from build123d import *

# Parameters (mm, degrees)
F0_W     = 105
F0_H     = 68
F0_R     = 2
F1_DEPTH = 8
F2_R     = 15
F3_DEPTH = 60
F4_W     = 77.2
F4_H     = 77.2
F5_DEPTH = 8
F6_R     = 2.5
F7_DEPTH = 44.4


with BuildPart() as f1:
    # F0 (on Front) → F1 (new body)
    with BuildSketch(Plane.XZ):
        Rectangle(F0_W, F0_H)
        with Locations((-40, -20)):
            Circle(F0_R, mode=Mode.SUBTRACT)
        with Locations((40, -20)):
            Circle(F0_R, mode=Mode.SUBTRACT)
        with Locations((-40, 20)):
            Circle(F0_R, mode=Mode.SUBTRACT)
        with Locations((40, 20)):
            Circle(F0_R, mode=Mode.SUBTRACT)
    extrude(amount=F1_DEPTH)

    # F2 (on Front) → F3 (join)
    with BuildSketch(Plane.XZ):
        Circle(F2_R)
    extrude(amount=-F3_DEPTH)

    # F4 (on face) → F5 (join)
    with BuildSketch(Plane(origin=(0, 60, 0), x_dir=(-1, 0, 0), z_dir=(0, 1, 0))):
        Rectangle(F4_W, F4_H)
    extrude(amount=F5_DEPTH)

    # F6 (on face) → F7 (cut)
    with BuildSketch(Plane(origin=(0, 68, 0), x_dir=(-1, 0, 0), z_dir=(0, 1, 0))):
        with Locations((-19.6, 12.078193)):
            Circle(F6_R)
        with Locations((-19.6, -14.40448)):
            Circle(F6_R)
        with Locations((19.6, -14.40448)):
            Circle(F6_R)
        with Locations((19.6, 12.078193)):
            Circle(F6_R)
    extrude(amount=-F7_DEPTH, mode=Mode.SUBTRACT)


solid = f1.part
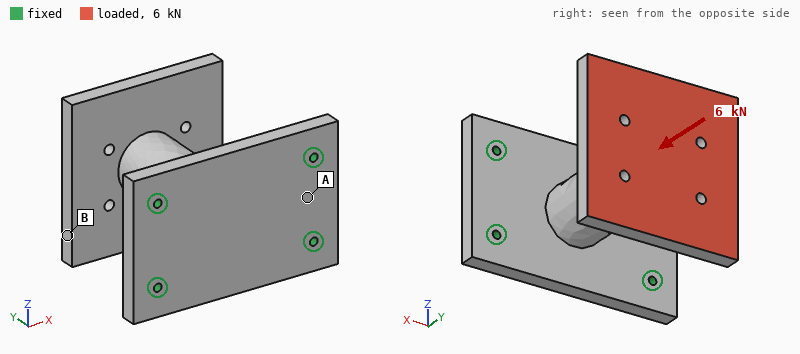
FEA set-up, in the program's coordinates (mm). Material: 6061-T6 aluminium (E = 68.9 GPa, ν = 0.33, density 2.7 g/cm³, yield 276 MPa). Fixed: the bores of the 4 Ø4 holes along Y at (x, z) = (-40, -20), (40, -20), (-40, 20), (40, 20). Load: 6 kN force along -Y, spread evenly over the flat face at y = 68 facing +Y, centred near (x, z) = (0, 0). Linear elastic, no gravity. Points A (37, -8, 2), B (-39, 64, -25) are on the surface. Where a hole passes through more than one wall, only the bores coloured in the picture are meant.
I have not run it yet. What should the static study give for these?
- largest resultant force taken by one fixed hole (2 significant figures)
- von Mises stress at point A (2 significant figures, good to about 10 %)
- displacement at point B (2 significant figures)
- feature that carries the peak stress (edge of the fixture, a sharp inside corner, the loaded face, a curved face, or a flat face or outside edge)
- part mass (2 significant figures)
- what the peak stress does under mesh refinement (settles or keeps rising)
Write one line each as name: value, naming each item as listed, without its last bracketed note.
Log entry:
largest resultant force taken by one fixed hole: 1.6 kN
von Mises stress at point A: 23 MPa
displacement at point B: 0.14 mm
feature that carries the peak stress: edge of the fixture
part mass: 390 g
what the peak stress does under mesh refinement: keeps rising
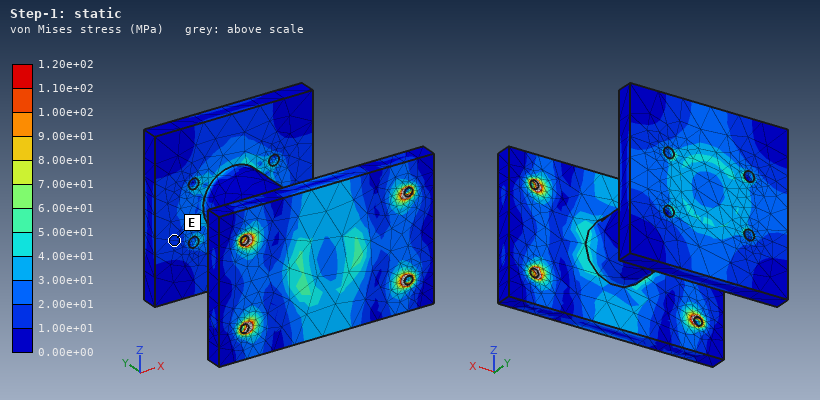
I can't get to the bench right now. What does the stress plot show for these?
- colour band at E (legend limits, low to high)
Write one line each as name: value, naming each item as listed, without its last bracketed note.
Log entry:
colour band at E: 1.00e+01 to 2.00e+01 MPa
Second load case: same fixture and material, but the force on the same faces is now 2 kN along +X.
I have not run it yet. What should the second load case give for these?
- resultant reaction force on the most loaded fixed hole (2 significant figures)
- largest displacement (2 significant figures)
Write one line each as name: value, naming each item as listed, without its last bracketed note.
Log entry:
resultant reaction force on the most loaded fixed hole: 1.3 kN
largest displacement: 0.29 mm
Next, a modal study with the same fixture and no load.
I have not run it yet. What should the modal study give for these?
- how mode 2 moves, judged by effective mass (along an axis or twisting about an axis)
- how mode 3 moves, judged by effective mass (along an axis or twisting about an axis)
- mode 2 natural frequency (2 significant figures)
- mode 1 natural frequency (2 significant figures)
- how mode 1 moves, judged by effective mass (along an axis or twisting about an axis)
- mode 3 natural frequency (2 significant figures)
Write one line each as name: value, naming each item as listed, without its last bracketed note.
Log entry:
how mode 2 moves, judged by effective mass: along X
how mode 3 moves, judged by effective mass: twisting about Y
mode 2 natural frequency: 1200 Hz
mode 1 natural frequency: 910 Hz
how mode 1 moves, judged by effective mass: along Z
mode 3 natural frequency: 2400 Hz
